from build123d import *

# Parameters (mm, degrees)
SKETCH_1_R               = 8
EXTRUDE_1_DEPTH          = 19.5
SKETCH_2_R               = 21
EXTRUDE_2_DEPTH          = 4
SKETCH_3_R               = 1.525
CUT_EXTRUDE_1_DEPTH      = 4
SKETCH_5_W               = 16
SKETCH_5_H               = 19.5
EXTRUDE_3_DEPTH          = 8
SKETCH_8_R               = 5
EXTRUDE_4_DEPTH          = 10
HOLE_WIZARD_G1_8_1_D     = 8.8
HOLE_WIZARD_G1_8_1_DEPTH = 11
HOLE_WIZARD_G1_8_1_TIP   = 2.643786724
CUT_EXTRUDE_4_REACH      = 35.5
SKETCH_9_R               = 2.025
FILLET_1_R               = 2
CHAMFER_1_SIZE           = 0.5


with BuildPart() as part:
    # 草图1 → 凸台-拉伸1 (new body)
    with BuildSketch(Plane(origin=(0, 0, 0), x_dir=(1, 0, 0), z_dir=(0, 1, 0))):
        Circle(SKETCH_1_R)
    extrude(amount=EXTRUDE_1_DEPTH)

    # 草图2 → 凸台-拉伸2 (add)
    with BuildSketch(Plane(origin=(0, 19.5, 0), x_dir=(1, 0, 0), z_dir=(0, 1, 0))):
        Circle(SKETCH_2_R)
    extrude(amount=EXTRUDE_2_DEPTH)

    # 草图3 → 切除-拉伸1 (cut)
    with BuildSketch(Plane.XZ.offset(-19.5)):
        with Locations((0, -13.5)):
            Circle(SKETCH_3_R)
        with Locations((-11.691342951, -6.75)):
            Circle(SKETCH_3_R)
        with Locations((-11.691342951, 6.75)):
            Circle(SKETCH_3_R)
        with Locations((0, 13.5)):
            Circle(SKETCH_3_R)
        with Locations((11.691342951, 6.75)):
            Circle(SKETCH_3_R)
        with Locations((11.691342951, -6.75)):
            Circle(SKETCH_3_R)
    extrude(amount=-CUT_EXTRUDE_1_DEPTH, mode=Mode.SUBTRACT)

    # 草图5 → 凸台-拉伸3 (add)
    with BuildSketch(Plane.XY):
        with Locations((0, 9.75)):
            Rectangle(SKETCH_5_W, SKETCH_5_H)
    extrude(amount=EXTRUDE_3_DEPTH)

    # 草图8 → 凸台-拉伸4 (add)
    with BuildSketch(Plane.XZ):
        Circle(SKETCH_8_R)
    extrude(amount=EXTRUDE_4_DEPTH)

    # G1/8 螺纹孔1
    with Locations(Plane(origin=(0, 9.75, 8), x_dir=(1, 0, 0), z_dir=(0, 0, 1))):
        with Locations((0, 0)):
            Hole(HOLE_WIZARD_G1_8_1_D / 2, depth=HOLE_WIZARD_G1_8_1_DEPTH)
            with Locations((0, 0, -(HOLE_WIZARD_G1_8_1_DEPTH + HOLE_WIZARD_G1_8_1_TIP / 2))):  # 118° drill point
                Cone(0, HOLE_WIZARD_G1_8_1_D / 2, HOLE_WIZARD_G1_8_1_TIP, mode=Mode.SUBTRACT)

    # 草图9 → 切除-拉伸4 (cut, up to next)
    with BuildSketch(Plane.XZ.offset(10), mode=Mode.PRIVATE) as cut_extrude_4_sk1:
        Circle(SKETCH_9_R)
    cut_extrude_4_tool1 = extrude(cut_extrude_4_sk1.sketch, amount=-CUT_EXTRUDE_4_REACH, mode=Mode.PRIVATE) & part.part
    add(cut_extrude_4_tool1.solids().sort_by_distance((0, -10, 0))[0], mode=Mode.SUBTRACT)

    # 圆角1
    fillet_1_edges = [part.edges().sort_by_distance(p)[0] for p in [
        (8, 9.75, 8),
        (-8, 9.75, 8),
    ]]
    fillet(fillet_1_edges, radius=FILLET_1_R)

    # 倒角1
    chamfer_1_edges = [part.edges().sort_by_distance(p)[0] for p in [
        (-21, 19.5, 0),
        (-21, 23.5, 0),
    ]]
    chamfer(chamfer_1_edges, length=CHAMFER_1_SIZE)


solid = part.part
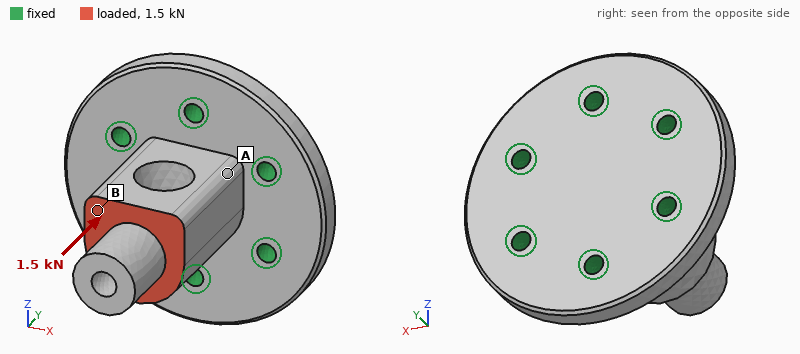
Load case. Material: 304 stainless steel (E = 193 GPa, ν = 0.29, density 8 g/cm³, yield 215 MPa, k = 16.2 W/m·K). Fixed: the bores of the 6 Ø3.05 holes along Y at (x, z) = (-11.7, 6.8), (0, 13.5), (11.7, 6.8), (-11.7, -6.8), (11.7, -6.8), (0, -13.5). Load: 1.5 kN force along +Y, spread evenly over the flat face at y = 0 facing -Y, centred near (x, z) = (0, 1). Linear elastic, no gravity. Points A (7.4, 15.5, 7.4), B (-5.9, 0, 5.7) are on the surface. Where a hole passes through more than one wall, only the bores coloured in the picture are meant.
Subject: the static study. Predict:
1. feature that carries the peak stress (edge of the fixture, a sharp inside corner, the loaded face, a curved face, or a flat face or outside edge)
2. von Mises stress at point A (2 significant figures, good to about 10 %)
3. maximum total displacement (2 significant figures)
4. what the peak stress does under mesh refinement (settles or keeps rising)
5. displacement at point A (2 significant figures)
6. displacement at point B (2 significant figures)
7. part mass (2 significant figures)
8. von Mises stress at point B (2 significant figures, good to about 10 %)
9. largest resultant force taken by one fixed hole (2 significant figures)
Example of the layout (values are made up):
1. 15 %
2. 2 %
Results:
1. edge of the fixture
2. 19 MPa
3. 2.9 µm
4. keeps rising
5. 1.3 µm
6. 2.5 µm
7. 77 g
8. 10.0 MPa
9. 320 N
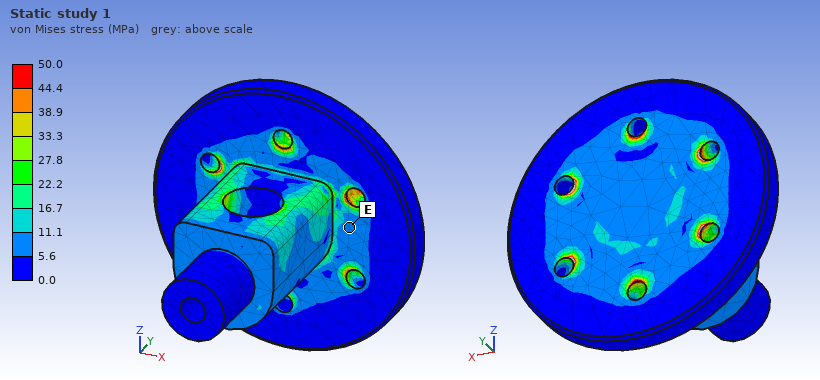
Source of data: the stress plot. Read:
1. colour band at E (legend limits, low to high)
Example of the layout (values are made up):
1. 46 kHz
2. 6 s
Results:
1. 5.6 to 11.1 MPa
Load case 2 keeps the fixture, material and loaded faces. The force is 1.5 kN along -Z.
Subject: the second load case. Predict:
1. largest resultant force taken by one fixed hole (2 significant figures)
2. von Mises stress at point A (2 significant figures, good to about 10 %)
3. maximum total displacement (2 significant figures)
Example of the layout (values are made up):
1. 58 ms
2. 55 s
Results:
1. 980 N
2. 63 MPa
3. 27 µm
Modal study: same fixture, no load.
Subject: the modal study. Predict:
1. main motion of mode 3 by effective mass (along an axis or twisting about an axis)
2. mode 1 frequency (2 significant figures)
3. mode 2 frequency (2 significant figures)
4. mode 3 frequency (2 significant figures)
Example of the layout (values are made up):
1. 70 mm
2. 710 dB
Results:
1. along Y
2. 11 kHz
3. 11 kHz
4. 24 kHz
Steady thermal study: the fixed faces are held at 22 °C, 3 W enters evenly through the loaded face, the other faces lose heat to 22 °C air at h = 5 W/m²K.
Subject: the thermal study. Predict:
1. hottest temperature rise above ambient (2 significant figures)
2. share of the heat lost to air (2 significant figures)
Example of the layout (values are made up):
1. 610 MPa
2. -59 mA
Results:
1. 28 K
2. 6.6 %
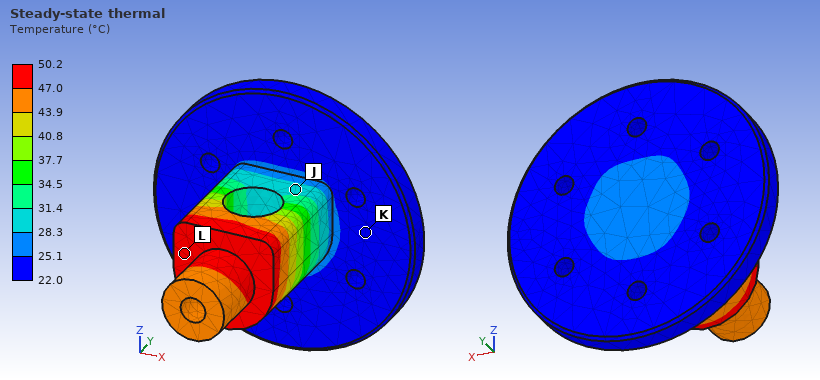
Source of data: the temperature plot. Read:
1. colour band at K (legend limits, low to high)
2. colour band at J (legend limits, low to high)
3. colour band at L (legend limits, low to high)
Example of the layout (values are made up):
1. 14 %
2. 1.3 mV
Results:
1. 22.0 to 25.1 °C
2. 28.3 to 31.4 °C
3. 47.0 to 50.2 °C
